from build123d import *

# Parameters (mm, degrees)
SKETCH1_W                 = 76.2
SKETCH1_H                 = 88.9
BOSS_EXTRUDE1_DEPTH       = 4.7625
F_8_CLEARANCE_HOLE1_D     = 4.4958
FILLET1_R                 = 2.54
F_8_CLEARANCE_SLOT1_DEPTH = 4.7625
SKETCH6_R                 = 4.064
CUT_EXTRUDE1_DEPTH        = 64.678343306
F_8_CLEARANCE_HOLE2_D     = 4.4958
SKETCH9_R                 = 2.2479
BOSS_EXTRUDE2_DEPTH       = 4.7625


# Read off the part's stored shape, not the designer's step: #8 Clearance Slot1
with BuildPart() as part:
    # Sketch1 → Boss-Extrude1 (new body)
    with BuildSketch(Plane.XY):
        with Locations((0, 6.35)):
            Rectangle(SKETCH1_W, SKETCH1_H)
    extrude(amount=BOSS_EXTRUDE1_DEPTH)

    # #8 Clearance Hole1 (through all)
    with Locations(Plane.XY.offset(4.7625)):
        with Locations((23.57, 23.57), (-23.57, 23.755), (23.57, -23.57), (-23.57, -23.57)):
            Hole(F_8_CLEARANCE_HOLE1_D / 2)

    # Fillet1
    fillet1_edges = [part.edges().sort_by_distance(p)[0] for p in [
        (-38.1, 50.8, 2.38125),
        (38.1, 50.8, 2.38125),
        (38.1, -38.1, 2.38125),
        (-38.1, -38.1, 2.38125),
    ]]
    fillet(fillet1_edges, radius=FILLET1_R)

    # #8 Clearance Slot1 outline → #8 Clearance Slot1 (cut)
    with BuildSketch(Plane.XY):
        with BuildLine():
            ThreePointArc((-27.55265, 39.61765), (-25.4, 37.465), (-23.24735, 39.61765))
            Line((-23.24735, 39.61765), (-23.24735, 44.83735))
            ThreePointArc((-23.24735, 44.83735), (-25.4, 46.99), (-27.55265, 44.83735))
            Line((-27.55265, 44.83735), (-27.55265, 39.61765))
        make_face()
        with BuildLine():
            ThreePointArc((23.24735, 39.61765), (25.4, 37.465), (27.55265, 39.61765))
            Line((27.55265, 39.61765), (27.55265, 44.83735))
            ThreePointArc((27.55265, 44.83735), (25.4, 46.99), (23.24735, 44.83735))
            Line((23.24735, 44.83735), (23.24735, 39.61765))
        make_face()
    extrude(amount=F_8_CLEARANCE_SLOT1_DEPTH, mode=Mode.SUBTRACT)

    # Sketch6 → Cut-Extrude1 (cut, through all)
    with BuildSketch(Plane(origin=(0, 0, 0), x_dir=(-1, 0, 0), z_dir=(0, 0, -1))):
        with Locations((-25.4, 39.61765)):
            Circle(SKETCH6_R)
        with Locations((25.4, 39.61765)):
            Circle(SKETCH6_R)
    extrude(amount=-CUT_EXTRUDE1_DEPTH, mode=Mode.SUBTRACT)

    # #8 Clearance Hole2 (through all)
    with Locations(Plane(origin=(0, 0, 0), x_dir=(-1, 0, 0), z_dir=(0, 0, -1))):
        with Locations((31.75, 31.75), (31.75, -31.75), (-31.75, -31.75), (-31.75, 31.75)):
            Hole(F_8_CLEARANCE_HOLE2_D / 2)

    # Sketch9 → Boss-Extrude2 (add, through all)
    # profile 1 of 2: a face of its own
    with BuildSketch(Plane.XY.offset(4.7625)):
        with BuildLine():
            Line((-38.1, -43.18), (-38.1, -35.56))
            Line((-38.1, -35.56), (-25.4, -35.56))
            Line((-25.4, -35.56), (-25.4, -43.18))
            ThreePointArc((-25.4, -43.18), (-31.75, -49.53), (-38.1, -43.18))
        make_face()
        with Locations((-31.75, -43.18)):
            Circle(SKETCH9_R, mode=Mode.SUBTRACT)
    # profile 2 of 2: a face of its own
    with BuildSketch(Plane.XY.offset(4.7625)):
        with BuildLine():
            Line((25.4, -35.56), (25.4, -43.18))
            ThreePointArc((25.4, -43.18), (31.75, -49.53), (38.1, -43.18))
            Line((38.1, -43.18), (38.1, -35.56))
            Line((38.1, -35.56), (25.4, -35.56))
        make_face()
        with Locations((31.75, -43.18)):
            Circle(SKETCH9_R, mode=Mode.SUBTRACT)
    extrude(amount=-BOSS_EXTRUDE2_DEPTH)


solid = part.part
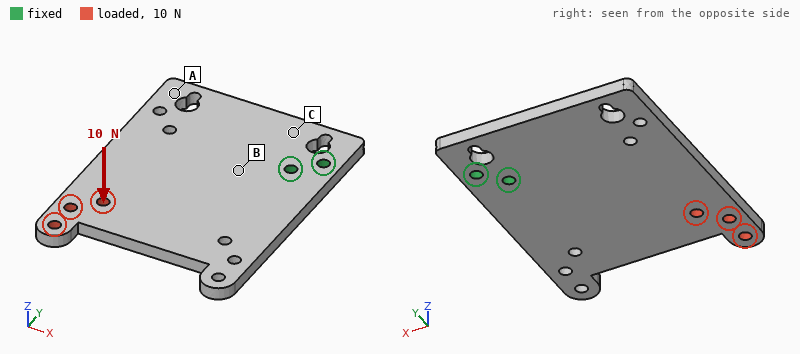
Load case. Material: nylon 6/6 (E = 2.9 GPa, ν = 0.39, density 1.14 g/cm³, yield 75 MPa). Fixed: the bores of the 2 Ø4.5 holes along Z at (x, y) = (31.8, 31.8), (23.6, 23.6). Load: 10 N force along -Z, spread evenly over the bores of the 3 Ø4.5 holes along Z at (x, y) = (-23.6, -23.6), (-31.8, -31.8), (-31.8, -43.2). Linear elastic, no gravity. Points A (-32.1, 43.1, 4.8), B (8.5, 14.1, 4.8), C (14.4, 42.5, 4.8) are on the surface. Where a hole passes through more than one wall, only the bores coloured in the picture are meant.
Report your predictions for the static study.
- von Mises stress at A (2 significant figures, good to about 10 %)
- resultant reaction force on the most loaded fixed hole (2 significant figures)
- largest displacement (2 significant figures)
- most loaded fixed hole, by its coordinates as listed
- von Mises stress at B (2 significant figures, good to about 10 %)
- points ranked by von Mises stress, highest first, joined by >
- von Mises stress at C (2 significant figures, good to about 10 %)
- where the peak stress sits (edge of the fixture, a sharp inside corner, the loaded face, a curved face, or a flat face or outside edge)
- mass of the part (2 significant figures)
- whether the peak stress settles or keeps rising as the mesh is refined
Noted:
0.61 MPa
40 N
1.4 mm
(23.6, 23.6)
2.3 MPa
B > C > A
1.5 MPa
edge of the fixture
37 g
keeps rising
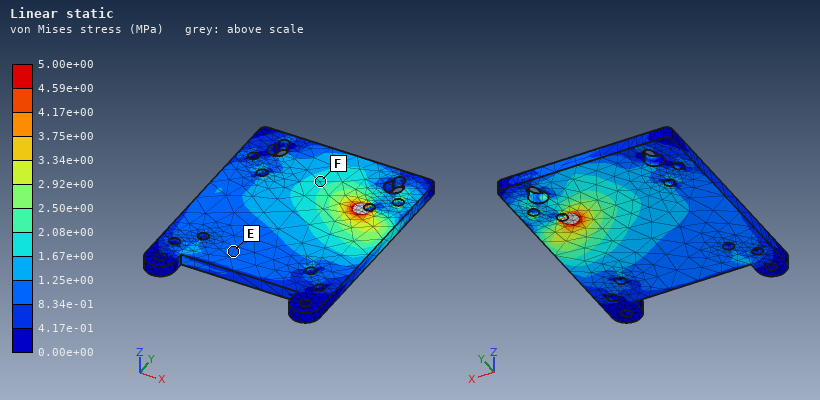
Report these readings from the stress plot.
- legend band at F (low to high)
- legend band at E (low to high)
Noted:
1.67e+00 to 2.08e+00 MPa
8.34e-01 to 1.25e+00 MPa
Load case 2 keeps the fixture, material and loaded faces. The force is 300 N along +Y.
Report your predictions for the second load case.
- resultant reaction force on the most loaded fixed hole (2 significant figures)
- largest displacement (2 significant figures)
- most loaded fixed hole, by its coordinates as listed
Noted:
1.2 kN
1.3 mm
(23.6, 23.6)
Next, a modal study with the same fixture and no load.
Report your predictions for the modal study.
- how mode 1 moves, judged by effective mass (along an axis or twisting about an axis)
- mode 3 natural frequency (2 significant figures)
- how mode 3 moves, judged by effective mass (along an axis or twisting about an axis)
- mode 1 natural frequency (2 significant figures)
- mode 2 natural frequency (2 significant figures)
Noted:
along Z
590 Hz
along Z
190 Hz
290 Hz
